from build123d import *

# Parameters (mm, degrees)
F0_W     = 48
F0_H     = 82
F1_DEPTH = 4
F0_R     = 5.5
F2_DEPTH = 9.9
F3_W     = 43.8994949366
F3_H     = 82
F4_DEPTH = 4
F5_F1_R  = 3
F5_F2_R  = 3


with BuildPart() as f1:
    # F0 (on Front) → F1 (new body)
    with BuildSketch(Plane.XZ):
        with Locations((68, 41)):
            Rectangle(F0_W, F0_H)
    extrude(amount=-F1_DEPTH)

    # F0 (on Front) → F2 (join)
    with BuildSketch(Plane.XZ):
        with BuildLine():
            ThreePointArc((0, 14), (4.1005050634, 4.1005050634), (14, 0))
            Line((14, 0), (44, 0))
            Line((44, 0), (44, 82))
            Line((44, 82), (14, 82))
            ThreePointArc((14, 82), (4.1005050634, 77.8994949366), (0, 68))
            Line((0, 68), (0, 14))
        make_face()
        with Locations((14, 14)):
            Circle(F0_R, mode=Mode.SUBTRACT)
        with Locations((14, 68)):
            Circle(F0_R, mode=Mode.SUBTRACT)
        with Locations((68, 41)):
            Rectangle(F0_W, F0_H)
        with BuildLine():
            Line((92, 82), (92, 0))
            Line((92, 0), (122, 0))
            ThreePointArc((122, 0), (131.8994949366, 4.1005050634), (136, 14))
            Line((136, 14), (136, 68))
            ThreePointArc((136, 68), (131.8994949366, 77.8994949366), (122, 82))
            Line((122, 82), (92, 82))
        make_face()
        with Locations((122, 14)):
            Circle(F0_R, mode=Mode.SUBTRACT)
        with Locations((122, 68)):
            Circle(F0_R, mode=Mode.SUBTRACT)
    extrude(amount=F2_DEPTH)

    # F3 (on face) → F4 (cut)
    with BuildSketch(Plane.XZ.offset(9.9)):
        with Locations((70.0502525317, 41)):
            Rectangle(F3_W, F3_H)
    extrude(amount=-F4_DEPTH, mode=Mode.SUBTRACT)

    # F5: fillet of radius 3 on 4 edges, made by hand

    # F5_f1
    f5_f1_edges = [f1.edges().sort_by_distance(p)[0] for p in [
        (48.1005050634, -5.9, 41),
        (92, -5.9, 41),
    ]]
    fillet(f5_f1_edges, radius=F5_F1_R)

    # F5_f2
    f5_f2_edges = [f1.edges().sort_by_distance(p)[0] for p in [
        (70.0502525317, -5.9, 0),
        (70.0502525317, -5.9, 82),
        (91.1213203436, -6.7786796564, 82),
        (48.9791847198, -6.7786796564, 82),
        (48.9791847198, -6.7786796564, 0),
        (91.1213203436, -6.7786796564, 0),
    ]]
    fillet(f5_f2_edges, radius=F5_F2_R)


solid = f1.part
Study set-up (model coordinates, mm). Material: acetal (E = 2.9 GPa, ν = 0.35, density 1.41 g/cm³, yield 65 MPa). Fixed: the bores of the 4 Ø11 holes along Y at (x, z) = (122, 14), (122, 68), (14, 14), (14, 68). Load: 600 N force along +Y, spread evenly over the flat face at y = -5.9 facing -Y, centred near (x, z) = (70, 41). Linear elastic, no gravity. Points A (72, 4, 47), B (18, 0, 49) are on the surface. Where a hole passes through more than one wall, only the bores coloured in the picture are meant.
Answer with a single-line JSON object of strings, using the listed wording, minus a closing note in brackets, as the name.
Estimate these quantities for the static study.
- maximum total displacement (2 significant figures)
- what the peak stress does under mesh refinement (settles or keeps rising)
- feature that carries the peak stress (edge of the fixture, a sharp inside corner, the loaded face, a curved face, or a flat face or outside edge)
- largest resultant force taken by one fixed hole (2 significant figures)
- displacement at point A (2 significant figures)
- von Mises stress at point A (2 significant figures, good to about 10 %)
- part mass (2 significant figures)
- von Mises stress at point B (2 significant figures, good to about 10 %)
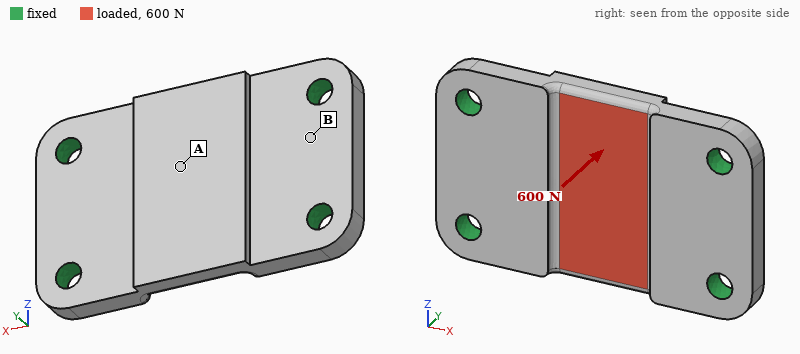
{"maximum total displacement": "0.15 mm", "what the peak stress does under mesh refinement": "keeps rising", "feature that carries the peak stress": "edge of the fixture", "largest resultant force taken by one fixed hole": "300 N", "displacement at point A": "0.15 mm", "von Mises stress at point A": "3.3 MPa", "part mass": "150 g", "von Mises stress at point B": "1.3 MPa"}
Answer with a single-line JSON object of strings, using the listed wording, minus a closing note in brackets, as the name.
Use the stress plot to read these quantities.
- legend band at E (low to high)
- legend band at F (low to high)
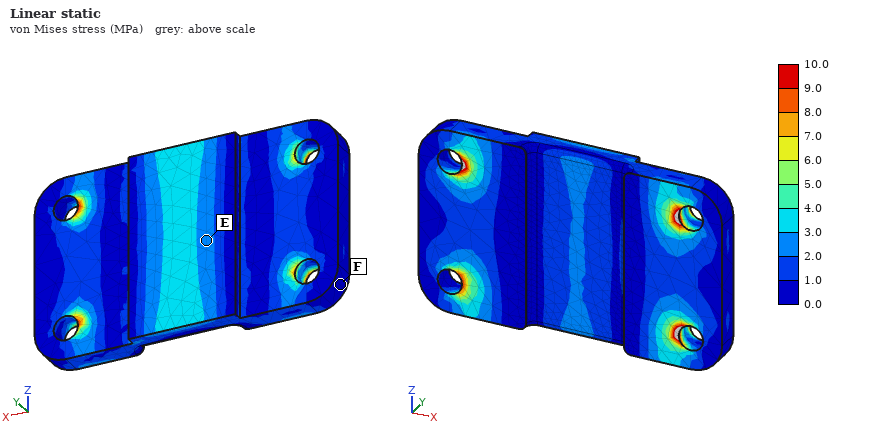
{"legend band at E": "2.0 to 3.0 MPa", "legend band at F": "0.0 to 1.0 MPa"}
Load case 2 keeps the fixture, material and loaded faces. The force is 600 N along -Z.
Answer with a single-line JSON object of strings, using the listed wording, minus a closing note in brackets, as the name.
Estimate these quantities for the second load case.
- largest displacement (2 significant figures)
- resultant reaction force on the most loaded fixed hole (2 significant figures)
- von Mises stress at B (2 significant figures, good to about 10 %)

{"largest displacement": "25 µm", "resultant reaction force on the most loaded fixed hole": "190 N", "von Mises stress at B": "0.48 MPa"}
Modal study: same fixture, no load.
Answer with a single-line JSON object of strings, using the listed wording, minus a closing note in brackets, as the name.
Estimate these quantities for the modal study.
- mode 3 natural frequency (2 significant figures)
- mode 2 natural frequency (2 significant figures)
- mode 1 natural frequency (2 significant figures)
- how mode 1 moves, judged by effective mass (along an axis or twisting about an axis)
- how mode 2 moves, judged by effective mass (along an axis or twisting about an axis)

{"mode 3 natural frequency": "2900 Hz", "mode 2 natural frequency": "1700 Hz", "mode 1 natural frequency": "1300 Hz", "how mode 1 moves, judged by effective mass": "along Y", "how mode 2 moves, judged by effective mass": "twisting about X"}
